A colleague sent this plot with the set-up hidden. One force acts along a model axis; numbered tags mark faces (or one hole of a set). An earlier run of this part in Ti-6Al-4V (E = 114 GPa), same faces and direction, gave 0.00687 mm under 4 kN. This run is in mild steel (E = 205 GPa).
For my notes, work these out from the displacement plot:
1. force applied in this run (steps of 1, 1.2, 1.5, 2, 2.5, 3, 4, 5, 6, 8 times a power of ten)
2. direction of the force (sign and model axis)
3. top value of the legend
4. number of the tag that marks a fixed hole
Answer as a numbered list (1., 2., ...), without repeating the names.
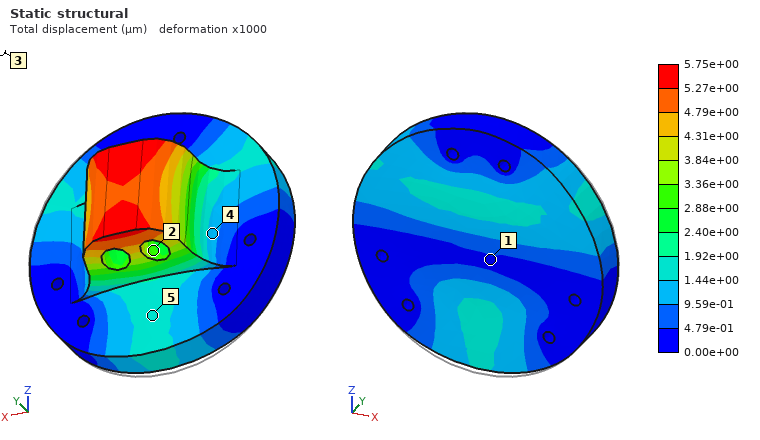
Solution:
1. 6 kN
2. +Z
3. 5.75e+00 µm
4. 3
